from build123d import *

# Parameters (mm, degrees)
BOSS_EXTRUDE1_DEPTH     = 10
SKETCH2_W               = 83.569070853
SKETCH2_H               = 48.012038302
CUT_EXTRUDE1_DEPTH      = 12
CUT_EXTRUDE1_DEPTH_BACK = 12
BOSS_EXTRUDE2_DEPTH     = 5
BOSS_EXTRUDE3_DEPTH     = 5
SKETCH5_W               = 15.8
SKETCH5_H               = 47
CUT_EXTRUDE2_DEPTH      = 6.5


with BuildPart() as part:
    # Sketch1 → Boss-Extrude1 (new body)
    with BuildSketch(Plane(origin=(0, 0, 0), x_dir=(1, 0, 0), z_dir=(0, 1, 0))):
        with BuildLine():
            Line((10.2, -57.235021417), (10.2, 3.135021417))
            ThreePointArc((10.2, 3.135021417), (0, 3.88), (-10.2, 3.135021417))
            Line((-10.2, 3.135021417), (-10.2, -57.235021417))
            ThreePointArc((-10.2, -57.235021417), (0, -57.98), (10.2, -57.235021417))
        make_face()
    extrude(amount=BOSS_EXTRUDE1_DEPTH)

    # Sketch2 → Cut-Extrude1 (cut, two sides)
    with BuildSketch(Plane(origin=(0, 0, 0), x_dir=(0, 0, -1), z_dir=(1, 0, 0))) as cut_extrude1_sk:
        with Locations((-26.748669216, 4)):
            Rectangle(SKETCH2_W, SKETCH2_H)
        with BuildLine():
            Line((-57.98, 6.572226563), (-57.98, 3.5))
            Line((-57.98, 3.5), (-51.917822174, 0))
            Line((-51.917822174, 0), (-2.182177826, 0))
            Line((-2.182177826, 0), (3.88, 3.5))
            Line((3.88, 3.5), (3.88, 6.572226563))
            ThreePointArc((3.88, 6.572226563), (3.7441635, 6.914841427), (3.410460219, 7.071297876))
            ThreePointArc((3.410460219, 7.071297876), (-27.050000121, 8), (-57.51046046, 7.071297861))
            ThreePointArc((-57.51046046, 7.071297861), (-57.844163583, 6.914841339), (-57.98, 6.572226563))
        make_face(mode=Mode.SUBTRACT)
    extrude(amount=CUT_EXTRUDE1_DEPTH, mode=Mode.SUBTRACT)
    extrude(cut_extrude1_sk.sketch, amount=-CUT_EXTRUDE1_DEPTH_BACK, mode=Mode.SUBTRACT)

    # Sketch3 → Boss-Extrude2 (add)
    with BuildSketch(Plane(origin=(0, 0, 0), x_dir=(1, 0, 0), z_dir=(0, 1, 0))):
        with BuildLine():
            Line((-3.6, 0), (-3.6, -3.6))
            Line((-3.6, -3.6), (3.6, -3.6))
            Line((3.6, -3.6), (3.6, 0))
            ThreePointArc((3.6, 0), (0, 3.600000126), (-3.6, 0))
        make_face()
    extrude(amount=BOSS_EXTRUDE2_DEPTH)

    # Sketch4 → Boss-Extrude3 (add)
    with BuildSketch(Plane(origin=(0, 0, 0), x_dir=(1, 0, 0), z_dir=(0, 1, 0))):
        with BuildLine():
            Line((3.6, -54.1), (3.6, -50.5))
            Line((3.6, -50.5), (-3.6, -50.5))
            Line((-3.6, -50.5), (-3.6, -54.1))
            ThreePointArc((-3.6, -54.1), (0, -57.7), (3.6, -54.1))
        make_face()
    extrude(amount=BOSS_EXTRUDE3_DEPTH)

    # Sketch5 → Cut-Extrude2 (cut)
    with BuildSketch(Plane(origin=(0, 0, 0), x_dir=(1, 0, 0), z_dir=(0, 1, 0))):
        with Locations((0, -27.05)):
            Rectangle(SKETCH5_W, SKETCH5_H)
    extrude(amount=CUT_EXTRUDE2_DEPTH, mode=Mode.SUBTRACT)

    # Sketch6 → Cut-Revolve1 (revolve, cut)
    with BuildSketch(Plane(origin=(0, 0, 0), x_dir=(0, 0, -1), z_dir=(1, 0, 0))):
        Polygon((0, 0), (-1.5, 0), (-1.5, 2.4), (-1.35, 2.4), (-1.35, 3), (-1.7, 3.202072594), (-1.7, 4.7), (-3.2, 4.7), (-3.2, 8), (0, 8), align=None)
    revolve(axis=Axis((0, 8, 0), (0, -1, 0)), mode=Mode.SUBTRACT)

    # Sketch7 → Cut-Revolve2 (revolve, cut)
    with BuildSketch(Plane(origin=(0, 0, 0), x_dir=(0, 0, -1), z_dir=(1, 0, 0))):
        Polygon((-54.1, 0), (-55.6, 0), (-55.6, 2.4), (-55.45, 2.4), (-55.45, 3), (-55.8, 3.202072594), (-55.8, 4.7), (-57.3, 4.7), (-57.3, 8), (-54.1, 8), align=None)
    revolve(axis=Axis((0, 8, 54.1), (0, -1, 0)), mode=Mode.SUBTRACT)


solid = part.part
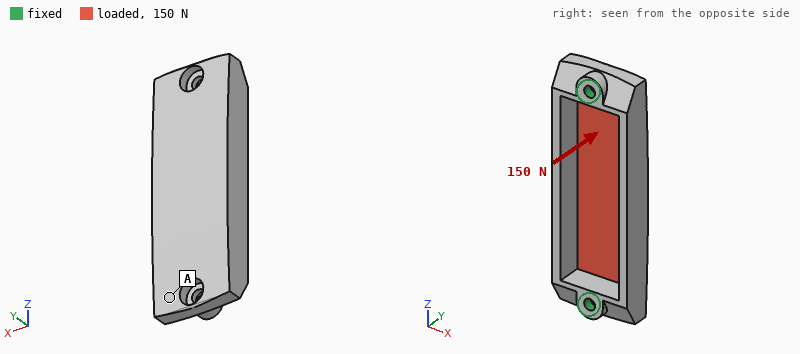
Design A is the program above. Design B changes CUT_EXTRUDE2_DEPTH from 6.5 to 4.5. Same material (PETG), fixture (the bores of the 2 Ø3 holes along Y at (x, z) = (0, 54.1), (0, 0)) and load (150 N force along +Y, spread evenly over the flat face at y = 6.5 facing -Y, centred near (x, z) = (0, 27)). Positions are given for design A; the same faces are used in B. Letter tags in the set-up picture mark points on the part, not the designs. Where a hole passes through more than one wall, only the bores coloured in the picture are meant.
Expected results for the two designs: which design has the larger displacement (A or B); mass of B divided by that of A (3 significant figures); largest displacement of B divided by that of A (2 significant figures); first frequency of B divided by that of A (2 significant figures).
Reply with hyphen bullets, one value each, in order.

- A
- 1.35
- 0.47
- 0.97
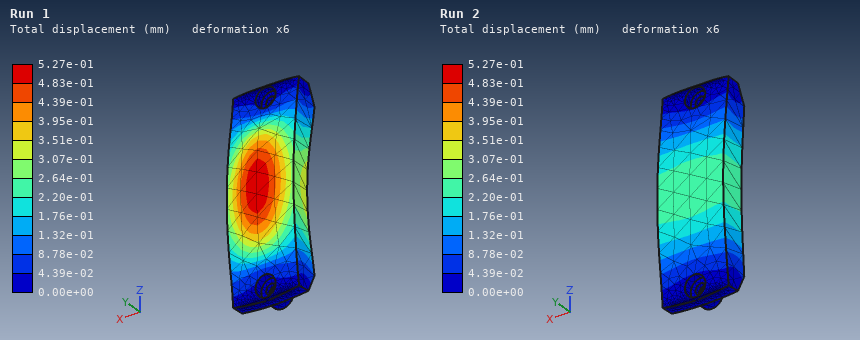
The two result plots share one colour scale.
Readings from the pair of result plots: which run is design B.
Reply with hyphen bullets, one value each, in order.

- Run 2
